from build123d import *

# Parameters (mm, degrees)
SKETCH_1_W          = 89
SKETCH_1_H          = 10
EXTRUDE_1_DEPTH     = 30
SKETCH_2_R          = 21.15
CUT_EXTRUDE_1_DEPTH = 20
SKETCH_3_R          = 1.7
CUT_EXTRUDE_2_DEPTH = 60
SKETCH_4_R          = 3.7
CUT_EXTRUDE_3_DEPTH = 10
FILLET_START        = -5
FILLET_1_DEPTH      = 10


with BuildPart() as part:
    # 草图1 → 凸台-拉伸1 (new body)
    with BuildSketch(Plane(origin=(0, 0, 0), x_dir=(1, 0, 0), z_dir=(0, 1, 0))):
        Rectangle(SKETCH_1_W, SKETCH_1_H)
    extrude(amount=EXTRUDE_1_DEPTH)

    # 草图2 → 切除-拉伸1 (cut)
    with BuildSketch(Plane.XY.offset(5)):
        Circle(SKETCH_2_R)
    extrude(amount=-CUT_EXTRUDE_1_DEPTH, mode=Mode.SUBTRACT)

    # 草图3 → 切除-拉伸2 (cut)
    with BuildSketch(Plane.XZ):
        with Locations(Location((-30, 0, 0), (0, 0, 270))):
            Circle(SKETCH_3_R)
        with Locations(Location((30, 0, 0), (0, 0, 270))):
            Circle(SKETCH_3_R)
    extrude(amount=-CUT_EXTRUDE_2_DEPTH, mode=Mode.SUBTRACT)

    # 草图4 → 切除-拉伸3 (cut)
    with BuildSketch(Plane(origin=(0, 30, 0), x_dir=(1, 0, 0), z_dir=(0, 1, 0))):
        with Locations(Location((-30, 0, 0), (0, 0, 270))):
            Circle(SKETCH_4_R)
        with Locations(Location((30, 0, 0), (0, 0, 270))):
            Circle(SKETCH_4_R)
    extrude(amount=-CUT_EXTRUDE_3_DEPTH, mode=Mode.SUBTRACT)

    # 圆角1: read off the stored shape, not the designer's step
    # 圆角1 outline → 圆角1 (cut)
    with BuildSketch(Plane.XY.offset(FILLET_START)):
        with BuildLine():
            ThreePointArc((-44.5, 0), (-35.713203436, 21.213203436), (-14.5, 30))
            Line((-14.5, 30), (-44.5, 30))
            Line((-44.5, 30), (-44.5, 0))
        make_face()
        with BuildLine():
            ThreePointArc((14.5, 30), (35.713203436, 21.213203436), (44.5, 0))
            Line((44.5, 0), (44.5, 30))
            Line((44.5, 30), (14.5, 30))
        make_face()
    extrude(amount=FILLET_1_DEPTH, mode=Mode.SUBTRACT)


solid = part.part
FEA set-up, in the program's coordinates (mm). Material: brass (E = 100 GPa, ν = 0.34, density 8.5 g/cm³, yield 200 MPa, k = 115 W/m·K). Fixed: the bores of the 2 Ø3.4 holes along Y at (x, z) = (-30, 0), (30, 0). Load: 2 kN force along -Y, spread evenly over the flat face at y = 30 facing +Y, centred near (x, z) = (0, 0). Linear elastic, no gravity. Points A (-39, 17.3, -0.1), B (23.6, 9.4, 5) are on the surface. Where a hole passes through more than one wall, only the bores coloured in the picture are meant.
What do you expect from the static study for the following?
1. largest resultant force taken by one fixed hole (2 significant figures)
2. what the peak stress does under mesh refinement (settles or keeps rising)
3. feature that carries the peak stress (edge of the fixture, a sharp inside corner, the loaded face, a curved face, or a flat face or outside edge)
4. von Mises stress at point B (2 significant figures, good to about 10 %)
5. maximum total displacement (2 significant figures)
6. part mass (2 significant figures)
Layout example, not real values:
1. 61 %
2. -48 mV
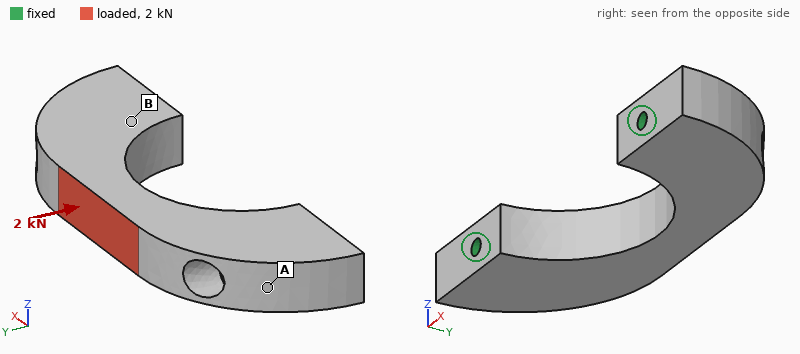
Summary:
1. 1.4 kN
2. keeps rising
3. edge of the fixture
4. 12 MPa
5. 8.8 µm
6. 130 g
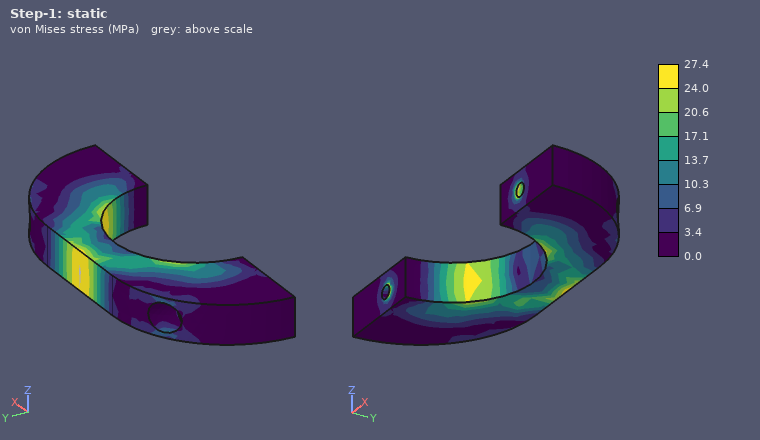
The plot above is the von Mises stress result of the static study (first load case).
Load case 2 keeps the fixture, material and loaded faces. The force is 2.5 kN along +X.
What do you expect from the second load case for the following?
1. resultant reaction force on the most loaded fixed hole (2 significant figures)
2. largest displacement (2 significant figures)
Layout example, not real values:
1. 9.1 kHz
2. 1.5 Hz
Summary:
1. 1.4 kN
2. 4.0 µm
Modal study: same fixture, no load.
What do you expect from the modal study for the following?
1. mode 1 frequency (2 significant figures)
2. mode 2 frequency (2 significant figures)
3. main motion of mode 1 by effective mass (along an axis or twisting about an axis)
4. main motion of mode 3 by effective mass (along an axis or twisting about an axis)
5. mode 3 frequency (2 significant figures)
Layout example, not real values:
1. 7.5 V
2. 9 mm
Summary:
1. 6700 Hz
2. 14 kHz
3. along Z
4. along Y
5. 15 kHz
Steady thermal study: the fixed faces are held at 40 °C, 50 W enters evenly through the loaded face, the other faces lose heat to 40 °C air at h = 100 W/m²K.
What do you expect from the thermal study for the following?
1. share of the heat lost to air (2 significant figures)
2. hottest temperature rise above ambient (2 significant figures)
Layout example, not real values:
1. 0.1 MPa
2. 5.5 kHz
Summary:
1. 11 %
2. 42 K
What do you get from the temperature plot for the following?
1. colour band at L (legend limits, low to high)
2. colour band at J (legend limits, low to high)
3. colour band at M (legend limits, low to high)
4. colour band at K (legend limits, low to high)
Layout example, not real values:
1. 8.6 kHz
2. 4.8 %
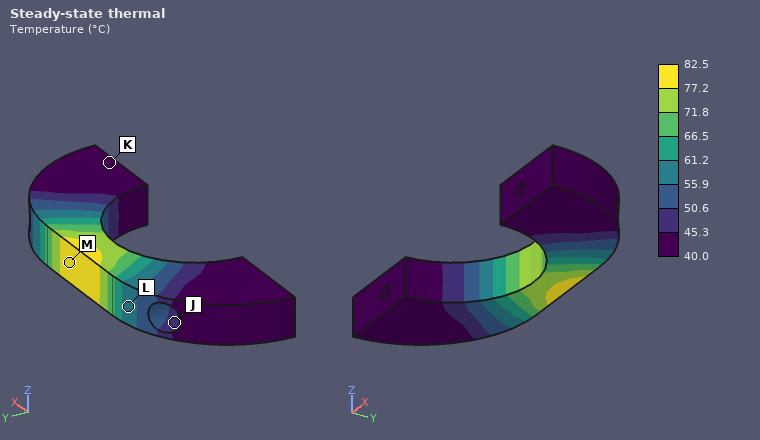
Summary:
1. 55.9 to 61.2 °C
2. 45.3 to 50.6 °C
3. 77.2 to 82.5 °C
4. 40.0 to 45.3 °C
